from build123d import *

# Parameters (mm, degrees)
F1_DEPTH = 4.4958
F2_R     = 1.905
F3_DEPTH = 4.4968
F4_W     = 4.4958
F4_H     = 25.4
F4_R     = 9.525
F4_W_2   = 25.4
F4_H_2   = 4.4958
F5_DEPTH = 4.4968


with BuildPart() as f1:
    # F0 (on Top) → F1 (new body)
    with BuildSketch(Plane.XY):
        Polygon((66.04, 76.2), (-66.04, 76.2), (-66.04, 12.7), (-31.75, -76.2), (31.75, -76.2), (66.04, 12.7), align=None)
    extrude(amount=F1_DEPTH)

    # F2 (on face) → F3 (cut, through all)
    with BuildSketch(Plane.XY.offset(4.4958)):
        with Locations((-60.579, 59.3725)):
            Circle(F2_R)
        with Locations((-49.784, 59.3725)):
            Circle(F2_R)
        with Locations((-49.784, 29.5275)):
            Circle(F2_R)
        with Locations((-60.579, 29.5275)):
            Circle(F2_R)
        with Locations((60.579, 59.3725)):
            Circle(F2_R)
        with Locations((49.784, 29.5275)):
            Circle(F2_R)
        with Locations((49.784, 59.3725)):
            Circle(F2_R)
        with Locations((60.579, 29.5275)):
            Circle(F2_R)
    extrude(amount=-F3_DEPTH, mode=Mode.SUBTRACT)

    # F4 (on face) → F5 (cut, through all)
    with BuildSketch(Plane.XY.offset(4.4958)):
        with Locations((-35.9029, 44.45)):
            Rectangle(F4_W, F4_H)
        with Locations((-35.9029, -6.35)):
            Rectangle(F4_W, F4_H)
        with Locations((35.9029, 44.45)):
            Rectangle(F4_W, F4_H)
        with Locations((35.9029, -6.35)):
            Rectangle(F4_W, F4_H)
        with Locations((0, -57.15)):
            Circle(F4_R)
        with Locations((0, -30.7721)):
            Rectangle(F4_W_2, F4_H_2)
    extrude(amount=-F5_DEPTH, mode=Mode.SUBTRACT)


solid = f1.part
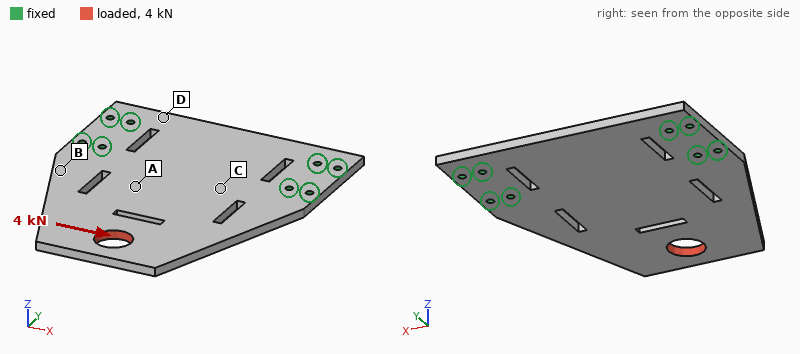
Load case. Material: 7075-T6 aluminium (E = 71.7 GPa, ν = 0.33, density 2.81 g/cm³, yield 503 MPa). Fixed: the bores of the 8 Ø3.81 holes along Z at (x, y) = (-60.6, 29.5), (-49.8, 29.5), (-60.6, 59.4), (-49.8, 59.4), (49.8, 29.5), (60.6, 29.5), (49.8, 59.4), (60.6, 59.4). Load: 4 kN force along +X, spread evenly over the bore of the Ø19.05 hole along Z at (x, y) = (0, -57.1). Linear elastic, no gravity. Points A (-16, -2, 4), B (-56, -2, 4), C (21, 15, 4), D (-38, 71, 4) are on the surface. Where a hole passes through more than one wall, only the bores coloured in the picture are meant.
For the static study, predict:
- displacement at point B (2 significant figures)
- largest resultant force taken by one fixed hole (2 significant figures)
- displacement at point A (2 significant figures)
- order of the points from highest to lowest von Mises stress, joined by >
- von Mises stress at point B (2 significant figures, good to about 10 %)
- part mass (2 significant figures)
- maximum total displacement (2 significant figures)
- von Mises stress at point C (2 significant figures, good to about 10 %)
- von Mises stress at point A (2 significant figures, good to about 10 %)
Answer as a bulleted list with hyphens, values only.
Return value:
- 18 µm
- 1.8 kN
- 16 µm
- B > A > C > D
- 27 MPa
- 200 g
- 71 µm
- 10 MPa
- 17 MPa
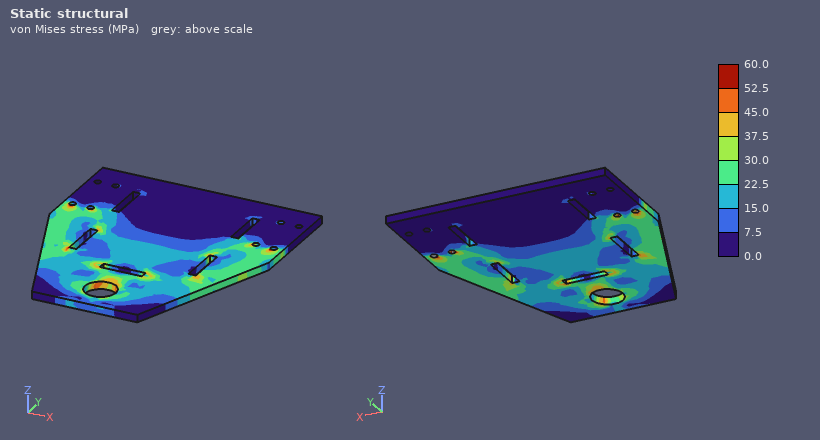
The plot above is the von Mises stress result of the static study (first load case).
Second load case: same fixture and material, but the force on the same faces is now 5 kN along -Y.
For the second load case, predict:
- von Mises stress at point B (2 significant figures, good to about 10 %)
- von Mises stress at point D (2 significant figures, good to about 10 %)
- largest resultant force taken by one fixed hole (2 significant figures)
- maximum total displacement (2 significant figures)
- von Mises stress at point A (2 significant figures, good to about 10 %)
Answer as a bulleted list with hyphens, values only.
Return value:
- 15 MPa
- 6.0 MPa
- 1.3 kN
- 36 µm
- 8.3 MPa
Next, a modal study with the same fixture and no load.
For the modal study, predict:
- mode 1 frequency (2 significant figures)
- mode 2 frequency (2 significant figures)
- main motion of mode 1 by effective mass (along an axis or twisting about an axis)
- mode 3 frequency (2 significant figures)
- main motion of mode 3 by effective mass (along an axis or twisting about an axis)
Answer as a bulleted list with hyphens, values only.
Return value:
- 370 Hz
- 1100 Hz
- along Z
- 1700 Hz
- along Z
